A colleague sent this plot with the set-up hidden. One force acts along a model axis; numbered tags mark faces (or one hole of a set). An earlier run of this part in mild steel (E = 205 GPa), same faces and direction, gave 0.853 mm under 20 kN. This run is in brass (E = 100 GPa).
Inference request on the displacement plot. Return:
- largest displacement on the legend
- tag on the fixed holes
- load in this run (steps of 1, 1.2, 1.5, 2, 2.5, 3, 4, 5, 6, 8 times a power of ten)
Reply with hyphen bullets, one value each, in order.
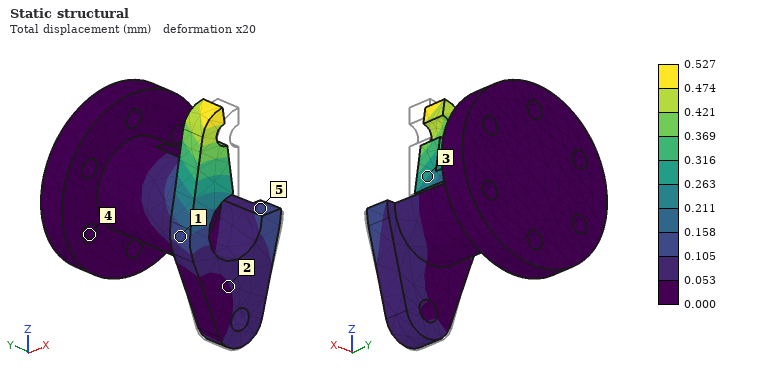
- 0.527 mm
- 4
- 6 kN
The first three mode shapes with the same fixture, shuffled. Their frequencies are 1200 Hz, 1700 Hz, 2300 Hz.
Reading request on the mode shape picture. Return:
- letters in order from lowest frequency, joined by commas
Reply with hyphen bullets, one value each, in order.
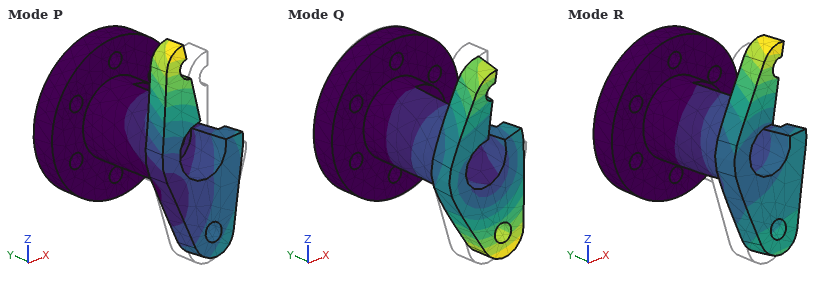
- P, R, Q
